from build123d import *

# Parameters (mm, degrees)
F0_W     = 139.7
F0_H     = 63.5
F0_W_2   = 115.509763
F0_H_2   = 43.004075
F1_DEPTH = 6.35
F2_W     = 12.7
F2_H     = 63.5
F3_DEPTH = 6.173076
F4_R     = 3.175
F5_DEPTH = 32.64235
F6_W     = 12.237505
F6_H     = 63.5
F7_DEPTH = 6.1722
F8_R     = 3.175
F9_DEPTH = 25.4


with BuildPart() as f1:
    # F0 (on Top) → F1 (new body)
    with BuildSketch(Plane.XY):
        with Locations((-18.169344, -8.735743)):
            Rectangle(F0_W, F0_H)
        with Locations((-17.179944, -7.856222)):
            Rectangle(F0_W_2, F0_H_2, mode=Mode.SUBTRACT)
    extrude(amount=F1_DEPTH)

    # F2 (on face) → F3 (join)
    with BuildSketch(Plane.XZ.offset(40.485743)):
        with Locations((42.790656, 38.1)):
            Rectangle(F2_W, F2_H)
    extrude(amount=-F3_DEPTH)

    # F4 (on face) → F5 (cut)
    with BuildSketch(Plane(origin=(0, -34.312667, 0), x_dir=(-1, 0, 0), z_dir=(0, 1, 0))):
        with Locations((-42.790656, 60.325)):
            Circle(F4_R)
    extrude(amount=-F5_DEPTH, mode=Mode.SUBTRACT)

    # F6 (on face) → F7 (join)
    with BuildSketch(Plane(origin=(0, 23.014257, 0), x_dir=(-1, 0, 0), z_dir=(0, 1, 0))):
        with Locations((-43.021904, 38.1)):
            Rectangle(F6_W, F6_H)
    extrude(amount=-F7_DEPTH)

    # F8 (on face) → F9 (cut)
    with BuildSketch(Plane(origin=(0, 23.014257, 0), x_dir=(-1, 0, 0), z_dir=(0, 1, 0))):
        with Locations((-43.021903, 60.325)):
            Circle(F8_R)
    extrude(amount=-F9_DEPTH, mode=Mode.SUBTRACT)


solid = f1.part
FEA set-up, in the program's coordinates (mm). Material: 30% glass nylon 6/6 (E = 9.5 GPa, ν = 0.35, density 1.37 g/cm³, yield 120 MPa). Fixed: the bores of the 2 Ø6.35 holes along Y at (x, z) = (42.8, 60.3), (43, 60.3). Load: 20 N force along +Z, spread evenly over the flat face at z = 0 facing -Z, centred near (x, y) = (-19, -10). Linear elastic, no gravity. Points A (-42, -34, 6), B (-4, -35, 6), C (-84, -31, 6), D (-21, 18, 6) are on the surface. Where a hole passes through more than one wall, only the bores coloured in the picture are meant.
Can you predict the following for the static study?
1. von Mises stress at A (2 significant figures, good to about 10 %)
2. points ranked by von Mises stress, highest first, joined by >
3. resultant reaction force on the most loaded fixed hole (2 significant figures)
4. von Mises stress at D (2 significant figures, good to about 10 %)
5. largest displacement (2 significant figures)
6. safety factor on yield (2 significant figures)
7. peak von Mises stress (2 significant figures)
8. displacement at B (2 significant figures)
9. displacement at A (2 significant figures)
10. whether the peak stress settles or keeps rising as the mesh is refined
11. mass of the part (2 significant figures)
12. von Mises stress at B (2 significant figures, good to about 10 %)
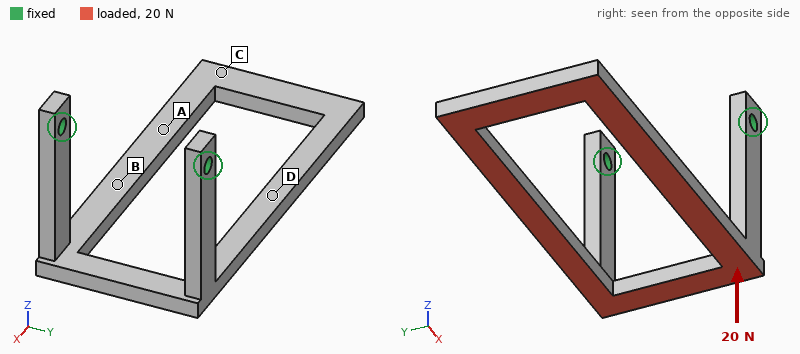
1.6 MPa
B > D > A > C
11 N
3.0 MPa
1.8 mm
14
8.6 MPa
0.42 mm
0.99 mm
settles
47 g
4.3 MPa
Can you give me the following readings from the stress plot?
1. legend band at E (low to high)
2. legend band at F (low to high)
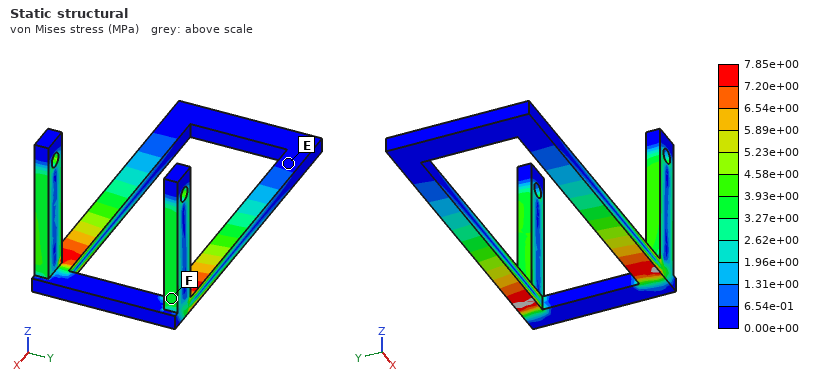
0.00e+00 to 6.54e-01 MPa
3.27e+00 to 3.93e+00 MPa
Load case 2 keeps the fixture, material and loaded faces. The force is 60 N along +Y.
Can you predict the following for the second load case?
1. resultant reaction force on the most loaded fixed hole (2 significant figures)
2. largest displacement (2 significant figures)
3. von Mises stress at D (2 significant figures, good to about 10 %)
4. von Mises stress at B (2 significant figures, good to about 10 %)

66 N
1.9 mm
2.6 MPa
3.0 MPa
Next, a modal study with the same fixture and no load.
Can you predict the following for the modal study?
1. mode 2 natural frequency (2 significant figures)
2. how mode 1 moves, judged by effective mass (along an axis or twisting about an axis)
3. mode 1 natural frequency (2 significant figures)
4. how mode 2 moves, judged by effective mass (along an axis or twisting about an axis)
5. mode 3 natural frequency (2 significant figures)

170 Hz
along Z
110 Hz
along Y
380 Hz
